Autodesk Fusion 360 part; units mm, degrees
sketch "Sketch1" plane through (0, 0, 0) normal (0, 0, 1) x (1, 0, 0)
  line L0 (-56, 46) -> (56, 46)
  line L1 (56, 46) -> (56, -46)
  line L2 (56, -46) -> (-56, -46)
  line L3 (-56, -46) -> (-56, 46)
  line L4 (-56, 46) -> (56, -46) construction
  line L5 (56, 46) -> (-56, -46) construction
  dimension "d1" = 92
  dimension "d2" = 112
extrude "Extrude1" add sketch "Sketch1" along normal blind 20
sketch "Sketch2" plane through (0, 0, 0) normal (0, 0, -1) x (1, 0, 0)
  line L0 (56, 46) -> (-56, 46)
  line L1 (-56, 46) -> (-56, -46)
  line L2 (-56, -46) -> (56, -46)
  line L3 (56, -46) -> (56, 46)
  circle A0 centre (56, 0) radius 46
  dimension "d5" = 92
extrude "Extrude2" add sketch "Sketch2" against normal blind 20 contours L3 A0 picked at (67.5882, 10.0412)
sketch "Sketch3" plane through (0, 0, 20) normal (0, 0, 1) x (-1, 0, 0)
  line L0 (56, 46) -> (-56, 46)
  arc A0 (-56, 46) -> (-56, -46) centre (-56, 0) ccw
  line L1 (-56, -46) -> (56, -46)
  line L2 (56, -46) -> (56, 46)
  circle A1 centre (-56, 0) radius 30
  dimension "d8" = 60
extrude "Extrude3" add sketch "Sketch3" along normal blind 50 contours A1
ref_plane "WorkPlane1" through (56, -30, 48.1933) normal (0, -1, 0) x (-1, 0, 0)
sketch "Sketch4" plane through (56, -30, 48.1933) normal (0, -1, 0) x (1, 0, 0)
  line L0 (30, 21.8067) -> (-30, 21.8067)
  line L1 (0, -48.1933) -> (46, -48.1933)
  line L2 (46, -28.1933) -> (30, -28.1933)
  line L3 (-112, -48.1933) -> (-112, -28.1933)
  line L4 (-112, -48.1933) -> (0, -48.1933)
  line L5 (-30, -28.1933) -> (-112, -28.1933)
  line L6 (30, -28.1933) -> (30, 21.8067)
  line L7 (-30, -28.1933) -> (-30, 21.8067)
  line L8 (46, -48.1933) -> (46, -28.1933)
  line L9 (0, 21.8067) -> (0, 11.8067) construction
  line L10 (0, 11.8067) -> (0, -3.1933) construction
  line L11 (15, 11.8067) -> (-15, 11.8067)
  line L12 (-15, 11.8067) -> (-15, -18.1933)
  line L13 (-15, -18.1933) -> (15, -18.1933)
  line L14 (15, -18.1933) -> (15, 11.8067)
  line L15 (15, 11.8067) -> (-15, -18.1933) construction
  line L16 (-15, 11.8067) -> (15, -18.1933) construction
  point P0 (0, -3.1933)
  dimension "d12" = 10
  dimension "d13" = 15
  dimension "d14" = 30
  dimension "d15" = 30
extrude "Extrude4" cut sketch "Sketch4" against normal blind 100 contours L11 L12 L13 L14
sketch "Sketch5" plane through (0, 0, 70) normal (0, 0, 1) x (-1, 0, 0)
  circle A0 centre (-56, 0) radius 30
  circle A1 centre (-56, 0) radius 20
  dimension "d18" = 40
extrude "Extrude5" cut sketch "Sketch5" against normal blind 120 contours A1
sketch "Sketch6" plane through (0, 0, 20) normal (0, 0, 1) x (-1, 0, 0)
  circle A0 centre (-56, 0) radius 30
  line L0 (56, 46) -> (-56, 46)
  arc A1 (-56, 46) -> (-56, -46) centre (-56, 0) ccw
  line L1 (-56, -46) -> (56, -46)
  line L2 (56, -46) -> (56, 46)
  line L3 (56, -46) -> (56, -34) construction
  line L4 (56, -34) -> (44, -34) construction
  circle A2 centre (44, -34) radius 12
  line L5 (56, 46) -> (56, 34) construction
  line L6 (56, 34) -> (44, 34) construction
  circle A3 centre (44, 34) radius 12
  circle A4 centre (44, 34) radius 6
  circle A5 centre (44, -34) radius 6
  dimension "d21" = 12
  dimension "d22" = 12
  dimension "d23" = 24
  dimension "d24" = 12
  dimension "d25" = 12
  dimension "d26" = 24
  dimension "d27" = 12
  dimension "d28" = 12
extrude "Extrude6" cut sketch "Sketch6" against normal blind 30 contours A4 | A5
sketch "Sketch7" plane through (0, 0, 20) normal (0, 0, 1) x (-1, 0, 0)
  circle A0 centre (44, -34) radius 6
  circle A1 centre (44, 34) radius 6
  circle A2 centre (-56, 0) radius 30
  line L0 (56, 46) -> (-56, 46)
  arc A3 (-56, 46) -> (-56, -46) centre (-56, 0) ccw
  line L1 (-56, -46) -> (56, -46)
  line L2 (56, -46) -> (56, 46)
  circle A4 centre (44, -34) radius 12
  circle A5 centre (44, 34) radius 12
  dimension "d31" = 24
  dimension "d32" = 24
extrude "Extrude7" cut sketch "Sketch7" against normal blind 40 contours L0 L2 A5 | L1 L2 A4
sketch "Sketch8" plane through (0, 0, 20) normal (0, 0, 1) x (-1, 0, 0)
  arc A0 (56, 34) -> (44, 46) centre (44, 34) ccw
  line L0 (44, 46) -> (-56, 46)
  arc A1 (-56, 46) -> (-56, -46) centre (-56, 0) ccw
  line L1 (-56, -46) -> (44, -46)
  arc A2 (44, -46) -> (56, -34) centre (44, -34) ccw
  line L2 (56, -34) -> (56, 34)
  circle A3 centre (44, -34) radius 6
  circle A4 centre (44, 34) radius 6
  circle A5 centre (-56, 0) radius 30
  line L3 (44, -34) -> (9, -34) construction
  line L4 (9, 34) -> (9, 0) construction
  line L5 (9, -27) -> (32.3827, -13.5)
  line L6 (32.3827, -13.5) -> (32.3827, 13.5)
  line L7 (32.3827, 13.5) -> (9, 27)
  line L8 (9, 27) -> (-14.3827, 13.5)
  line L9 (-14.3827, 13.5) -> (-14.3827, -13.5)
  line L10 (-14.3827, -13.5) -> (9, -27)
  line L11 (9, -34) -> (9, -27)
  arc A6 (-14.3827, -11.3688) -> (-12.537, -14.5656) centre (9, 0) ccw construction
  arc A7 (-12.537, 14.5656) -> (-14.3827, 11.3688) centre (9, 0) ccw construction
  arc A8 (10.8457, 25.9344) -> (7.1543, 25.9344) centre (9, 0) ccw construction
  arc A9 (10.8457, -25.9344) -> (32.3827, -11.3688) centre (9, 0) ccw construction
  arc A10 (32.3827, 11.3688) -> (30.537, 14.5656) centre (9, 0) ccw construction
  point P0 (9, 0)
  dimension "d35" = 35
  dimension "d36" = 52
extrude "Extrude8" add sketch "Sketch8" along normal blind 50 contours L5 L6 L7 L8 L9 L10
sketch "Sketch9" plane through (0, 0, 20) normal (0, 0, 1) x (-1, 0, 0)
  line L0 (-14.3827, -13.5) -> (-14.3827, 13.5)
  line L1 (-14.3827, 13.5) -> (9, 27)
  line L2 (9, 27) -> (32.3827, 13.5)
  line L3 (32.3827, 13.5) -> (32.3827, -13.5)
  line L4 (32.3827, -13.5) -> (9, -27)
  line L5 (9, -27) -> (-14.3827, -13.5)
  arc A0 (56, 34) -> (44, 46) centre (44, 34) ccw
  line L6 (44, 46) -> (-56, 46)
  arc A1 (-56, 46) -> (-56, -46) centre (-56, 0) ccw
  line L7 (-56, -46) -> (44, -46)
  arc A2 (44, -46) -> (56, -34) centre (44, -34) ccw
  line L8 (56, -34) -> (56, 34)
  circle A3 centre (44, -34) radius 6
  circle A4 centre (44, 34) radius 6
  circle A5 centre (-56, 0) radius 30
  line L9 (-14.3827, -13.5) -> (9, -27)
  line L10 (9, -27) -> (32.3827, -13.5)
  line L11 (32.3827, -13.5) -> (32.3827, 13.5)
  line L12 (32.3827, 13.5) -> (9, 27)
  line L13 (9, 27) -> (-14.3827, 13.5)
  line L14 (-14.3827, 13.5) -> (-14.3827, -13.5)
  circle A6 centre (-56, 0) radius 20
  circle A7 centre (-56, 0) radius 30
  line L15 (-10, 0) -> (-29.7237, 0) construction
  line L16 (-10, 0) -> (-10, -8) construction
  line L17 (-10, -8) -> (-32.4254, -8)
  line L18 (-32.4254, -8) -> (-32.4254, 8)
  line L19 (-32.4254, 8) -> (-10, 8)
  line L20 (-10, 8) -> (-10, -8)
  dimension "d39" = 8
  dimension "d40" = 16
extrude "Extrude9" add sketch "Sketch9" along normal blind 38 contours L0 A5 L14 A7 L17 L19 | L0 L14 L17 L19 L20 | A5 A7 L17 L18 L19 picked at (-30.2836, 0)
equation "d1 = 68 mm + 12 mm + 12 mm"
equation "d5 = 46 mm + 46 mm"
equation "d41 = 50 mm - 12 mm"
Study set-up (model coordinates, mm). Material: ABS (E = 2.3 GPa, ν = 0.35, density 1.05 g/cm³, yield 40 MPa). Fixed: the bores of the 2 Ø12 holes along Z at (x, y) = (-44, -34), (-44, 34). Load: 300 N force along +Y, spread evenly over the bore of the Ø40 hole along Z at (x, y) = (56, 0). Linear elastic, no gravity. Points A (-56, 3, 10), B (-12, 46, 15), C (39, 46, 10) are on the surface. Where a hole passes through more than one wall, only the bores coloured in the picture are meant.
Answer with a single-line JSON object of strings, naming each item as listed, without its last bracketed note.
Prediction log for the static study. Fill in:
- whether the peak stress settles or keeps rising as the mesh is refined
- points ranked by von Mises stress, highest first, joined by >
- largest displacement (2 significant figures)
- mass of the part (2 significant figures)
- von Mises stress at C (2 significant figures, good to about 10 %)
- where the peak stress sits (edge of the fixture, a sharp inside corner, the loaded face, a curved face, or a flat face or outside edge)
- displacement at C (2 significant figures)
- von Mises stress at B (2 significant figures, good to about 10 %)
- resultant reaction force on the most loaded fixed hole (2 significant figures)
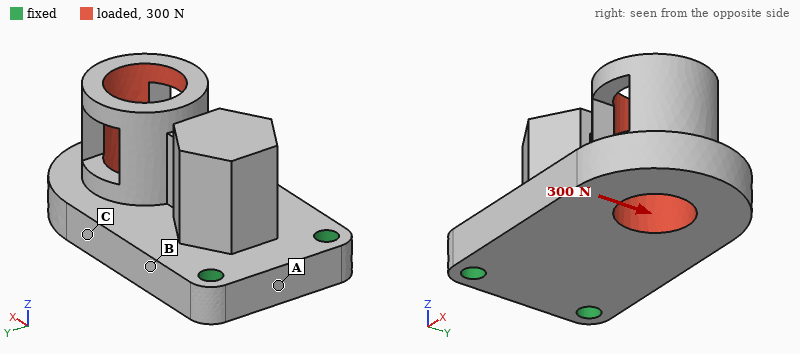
{"whether the peak stress settles or keeps rising as the mesh is refined": "keeps rising", "points ranked by von Mises stress, highest first, joined by >": "B > C > A", "largest displacement": "0.14 mm", "mass of the part": "420 g", "von Mises stress at C": "0.41 MPa", "where the peak stress sits": "edge of the fixture", "displacement at C": "0.055 mm", "von Mises stress at B": "0.64 MPa", "resultant reaction force on the most loaded fixed hole": "450 N"}
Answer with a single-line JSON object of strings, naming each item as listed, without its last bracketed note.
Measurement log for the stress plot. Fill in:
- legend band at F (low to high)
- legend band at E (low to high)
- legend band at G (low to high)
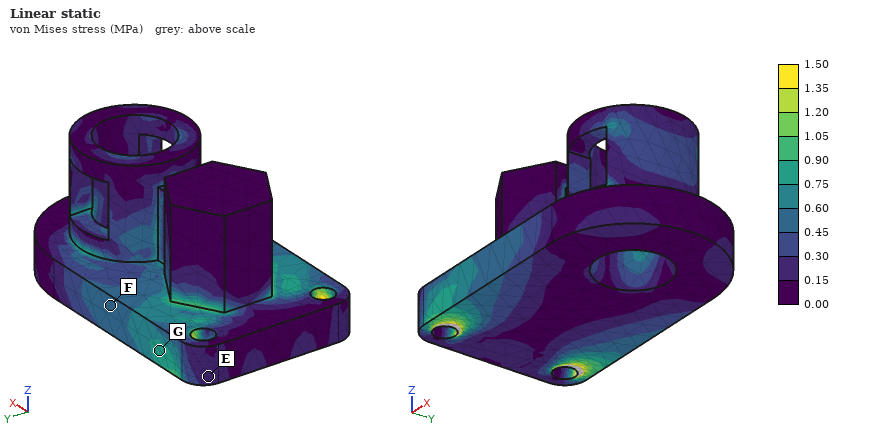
{"legend band at F": "0.45 to 0.60 MPa", "legend band at E": "0.15 to 0.30 MPa", "legend band at G": "0.75 to 0.90 MPa"}
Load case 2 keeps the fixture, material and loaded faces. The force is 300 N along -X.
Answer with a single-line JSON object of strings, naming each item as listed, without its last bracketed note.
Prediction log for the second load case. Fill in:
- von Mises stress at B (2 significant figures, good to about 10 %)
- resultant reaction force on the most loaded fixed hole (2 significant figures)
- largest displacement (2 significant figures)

{"von Mises stress at B": "0.48 MPa", "resultant reaction force on the most loaded fixed hole": "160 N", "largest displacement": "0.24 mm"}
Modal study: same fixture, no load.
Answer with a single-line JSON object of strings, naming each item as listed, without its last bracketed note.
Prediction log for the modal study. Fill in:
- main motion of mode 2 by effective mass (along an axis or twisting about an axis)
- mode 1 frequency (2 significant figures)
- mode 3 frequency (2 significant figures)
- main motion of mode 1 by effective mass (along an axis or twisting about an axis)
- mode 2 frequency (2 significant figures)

{"main motion of mode 2 by effective mass": "along Y", "mode 1 frequency": "240 Hz", "mode 3 frequency": "890 Hz", "main motion of mode 1 by effective mass": "along Z", "mode 2 frequency": "710 Hz"}
